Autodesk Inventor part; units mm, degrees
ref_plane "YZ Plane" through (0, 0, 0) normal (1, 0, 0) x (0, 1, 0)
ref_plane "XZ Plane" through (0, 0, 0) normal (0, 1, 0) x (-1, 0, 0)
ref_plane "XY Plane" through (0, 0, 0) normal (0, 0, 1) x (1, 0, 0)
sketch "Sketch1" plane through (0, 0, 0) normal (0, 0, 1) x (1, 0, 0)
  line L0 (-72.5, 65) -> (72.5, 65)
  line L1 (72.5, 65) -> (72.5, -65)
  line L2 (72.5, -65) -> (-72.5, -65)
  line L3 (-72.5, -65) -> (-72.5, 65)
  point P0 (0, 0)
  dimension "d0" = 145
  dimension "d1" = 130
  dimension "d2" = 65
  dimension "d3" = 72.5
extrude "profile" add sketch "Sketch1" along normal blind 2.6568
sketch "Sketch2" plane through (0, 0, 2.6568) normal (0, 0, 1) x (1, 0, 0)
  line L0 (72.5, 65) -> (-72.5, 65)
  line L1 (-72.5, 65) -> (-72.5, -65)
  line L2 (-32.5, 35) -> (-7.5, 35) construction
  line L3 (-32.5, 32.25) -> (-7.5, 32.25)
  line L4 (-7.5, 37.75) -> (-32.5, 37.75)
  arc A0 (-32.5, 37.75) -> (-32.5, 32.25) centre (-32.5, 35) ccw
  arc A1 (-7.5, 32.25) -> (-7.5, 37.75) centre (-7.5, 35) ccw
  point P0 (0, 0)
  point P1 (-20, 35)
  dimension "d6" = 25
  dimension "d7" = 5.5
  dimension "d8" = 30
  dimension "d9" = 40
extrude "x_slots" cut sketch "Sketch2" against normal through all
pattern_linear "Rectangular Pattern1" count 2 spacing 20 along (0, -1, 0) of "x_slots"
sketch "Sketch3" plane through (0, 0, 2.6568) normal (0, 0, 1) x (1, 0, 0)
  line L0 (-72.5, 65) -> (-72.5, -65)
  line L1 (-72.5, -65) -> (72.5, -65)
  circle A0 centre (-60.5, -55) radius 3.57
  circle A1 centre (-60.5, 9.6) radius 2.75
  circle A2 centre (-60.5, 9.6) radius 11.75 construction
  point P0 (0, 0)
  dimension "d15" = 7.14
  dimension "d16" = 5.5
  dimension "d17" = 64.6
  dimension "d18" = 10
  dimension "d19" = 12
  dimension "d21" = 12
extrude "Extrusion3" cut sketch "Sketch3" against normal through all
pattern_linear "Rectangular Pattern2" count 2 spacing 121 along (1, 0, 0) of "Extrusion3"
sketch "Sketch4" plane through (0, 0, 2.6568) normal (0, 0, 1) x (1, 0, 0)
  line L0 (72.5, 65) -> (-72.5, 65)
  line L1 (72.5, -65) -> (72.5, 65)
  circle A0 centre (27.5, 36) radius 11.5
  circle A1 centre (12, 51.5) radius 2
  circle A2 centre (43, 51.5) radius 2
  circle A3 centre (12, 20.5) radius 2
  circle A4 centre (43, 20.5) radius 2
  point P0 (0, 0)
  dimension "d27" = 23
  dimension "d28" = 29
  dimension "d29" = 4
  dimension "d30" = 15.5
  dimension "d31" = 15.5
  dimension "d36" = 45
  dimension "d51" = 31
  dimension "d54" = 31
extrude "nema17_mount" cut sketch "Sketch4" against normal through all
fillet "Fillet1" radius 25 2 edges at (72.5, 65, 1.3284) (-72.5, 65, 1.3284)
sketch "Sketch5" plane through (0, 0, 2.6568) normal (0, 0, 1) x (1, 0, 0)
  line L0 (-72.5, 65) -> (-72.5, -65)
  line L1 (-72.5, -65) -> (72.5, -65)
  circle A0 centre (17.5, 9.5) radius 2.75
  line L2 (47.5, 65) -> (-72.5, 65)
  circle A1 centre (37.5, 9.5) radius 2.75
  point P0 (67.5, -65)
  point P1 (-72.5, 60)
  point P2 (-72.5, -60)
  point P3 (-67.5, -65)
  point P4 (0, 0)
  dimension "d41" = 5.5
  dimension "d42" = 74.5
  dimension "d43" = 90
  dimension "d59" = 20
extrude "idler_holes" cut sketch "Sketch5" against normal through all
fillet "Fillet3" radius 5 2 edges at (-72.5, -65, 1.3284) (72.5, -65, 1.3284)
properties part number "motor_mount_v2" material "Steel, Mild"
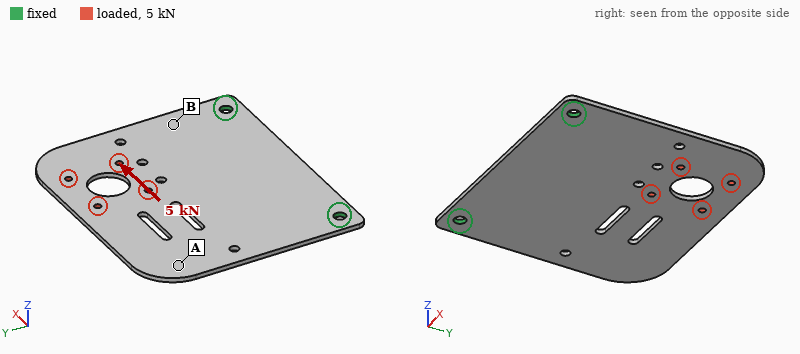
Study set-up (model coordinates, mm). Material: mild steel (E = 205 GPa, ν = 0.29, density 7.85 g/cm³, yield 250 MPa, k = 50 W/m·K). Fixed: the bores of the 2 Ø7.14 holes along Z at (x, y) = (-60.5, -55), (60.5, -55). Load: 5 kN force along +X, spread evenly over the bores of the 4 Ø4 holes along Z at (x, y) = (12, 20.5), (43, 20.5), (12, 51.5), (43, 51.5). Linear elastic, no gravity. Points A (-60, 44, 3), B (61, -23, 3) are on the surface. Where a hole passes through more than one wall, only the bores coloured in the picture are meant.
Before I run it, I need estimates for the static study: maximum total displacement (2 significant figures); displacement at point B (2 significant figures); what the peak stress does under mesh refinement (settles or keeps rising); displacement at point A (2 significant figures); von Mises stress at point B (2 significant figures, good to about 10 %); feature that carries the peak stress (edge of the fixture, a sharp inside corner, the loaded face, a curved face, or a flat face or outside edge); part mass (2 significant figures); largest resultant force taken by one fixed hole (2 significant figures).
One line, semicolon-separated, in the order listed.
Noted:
48 µm; 13 µm; keeps rising; 36 µm; 34 MPa; edge of the fixture; 370 g; 4.5 kN
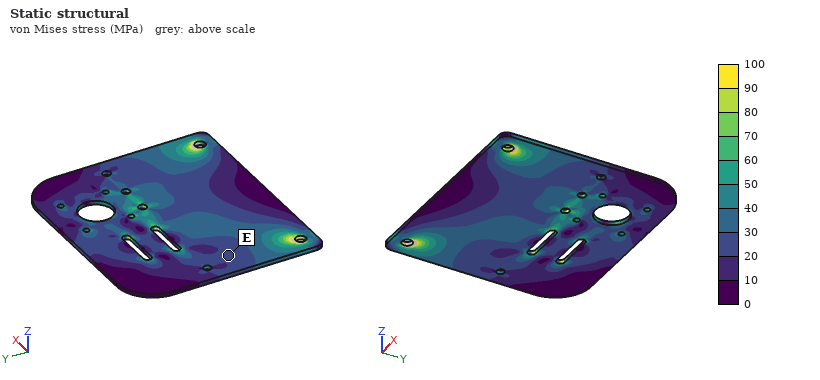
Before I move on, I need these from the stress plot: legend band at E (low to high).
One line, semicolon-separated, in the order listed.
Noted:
20 to 30 MPa
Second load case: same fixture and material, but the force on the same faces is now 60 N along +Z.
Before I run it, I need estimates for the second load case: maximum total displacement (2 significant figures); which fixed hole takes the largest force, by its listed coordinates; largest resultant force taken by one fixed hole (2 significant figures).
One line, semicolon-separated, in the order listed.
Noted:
0.76 mm; (60.5, -55); 44 N
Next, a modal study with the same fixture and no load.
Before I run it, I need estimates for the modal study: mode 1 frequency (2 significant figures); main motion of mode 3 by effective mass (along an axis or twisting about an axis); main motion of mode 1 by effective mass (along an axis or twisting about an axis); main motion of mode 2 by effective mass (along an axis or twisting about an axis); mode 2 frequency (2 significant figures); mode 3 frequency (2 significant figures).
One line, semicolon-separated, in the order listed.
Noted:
140 Hz; along Z; along Z; twisting about Y; 350 Hz; 740 Hz
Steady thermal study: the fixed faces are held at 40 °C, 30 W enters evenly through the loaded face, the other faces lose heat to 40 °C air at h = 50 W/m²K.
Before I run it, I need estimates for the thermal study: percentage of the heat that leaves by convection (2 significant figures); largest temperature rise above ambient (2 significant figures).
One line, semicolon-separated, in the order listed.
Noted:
94 %; 65 K
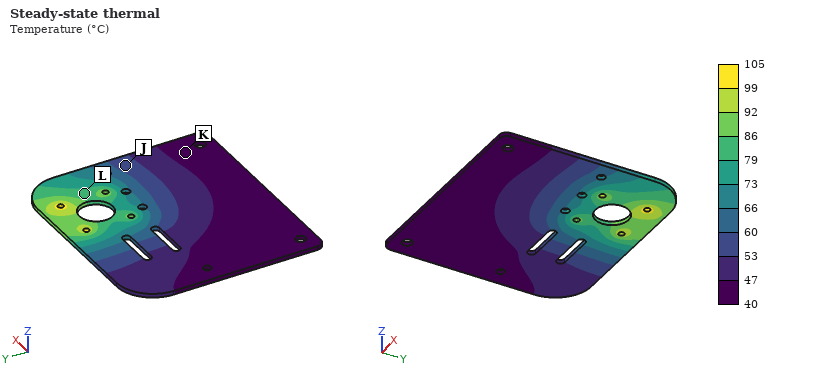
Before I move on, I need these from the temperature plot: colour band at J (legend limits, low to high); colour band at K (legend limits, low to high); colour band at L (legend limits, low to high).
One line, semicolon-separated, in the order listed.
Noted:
53 to 60 °C; 40 to 47 °C; 79 to 86 °C
